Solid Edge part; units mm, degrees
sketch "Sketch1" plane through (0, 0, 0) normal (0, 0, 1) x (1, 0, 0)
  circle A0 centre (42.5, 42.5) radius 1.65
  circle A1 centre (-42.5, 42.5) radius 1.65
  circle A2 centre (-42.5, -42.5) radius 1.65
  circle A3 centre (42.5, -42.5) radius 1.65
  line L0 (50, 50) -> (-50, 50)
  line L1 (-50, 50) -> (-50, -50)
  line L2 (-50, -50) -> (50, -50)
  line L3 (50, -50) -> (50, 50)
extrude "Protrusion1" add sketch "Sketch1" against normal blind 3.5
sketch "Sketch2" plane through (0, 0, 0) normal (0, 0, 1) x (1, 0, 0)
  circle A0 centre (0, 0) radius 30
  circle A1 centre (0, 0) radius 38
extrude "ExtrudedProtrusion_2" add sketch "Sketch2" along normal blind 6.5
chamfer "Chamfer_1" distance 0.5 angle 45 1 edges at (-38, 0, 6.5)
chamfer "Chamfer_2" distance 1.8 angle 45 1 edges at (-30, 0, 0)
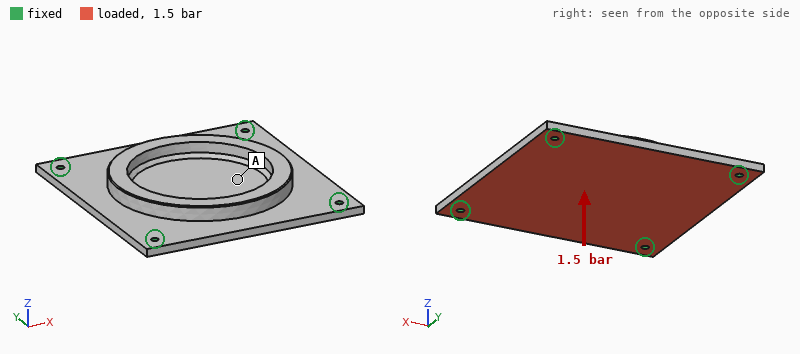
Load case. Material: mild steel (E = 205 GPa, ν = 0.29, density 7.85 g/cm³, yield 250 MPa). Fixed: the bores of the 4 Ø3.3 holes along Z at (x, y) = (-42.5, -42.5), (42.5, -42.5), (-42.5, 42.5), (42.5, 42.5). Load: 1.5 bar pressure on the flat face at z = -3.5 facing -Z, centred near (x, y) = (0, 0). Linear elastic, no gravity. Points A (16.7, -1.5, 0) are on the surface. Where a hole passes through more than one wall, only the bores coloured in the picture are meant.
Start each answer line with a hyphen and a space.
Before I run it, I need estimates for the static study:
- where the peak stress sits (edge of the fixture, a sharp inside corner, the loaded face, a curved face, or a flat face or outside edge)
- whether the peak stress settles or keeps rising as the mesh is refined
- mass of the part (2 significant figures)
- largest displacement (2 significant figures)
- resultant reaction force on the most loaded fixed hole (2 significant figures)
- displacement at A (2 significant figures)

- edge of the fixture
- keeps rising
- 360 g
- 34 µm
- 420 N
- 31 µm
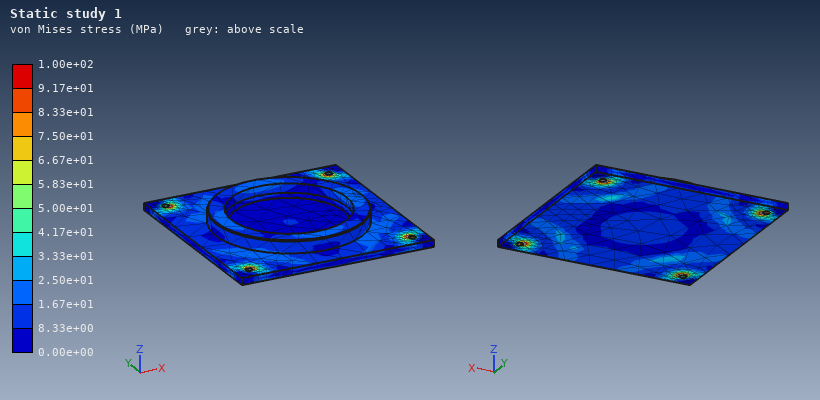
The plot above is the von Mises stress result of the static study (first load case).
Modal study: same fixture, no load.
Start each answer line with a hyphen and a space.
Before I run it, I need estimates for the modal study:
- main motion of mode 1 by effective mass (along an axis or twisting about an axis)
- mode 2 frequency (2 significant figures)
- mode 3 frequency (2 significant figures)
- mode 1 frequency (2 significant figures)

- along Z
- 3000 Hz
- 3000 Hz
- 2000 Hz
